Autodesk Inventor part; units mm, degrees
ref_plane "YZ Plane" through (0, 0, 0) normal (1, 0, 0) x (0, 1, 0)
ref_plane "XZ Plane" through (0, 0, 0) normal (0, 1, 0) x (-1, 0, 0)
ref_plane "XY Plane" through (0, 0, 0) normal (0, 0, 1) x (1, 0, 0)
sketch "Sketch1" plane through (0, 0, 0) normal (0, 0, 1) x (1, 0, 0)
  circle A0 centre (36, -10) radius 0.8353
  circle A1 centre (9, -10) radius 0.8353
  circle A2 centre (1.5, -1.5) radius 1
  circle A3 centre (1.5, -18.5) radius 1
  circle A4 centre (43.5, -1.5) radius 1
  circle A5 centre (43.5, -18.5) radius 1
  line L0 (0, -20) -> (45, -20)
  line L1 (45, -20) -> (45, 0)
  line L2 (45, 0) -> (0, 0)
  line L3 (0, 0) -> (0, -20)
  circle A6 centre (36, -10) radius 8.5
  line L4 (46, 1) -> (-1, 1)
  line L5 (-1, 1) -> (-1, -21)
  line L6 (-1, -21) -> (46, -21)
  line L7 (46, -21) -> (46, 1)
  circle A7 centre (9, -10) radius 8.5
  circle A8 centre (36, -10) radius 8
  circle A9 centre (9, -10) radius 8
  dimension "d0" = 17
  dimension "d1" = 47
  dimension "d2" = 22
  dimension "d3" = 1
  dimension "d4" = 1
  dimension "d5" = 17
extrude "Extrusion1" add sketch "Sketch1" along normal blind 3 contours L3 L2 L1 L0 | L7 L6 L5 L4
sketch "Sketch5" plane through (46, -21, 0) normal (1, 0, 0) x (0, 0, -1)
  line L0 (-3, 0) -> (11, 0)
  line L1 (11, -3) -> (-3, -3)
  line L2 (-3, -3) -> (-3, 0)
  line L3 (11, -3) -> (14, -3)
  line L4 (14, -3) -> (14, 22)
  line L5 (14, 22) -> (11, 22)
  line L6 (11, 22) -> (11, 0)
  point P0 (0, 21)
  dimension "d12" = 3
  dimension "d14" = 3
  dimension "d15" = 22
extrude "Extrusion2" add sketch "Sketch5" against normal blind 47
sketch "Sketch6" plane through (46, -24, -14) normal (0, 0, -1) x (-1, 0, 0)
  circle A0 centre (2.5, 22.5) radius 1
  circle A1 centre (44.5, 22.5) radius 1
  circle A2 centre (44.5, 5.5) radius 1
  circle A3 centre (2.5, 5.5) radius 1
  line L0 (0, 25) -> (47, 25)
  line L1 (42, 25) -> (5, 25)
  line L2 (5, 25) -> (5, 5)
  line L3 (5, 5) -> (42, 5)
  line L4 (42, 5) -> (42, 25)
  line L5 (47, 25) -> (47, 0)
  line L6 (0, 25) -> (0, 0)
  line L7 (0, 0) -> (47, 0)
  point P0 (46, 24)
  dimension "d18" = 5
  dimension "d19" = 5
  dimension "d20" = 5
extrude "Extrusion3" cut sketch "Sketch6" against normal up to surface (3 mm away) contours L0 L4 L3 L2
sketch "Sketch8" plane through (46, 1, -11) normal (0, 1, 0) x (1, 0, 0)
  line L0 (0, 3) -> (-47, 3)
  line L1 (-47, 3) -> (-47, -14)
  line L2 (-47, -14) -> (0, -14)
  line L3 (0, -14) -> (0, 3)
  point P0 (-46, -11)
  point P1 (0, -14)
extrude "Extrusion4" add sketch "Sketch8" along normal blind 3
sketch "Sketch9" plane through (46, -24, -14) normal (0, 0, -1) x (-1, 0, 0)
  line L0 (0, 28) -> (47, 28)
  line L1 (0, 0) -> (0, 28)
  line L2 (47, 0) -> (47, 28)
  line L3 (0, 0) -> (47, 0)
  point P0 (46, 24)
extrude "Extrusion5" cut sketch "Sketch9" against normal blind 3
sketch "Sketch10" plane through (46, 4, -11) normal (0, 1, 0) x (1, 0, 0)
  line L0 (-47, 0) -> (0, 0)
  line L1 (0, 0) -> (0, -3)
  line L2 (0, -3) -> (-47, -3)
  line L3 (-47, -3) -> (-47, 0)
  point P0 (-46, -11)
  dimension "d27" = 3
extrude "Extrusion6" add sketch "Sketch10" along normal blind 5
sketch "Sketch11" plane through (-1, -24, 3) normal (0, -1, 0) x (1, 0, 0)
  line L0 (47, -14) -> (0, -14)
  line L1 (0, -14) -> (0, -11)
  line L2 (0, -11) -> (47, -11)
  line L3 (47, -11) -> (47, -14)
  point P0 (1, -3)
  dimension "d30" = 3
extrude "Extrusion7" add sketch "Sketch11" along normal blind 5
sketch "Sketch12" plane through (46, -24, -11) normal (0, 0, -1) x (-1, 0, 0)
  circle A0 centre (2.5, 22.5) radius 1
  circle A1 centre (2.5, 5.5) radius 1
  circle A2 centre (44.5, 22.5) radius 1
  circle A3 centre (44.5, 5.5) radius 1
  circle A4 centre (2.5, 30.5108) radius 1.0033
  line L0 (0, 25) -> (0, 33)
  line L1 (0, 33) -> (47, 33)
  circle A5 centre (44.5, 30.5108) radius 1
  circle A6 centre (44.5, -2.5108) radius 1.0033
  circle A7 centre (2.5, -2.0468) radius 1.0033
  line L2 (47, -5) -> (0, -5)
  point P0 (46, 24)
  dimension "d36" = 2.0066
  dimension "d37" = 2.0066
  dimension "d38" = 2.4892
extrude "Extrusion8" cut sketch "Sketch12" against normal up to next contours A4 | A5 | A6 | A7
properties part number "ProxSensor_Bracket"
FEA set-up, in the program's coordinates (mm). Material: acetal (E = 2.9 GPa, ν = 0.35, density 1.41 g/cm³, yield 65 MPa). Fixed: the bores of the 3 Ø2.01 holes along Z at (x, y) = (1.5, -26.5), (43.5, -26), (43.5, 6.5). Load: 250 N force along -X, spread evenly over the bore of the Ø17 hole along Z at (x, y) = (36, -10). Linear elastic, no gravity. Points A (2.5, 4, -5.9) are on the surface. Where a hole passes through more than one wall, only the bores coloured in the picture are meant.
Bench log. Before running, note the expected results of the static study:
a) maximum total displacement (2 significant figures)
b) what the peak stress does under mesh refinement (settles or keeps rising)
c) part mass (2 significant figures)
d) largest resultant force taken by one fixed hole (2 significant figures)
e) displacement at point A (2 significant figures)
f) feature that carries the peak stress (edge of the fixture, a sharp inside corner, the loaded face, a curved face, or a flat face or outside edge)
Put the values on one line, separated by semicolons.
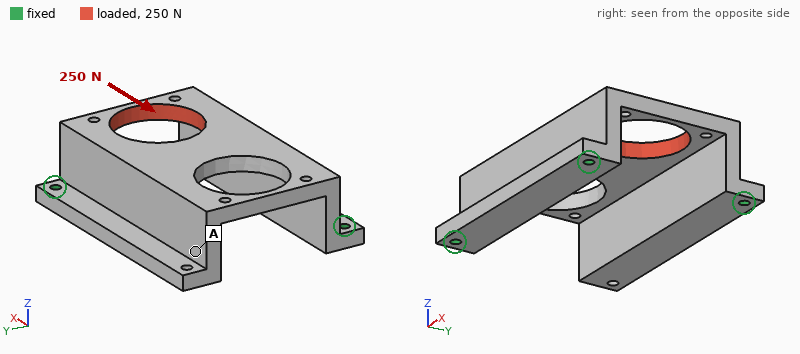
0.66 mm; keeps rising; 9.9 g; 120 N; 0.55 mm; edge of the fixture
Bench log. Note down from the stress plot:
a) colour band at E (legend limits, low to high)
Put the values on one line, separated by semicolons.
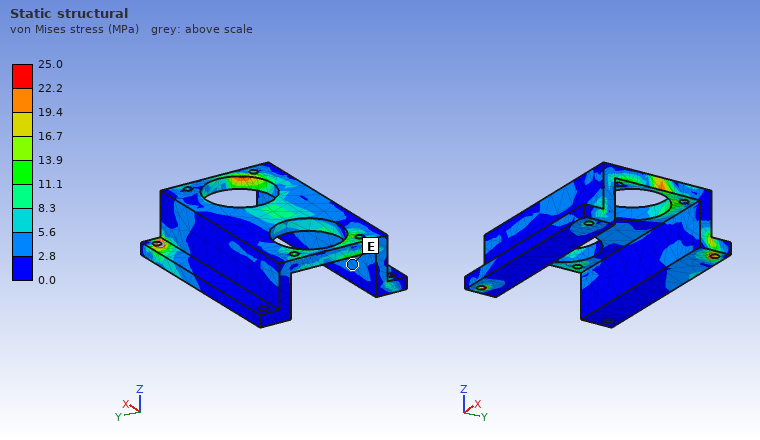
2.8 to 5.6 MPa
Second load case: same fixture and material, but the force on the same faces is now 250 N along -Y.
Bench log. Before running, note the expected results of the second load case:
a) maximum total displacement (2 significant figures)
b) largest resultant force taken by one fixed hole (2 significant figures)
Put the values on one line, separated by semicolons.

0.66 mm; 130 N
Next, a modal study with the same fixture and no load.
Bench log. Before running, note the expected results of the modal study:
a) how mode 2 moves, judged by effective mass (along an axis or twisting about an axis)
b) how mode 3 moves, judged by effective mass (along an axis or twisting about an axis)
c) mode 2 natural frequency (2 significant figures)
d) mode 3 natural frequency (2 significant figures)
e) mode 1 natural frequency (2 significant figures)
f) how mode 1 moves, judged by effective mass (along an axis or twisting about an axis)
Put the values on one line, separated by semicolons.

along Y; along Y; 1400 Hz; 2500 Hz; 810 Hz; along Z
